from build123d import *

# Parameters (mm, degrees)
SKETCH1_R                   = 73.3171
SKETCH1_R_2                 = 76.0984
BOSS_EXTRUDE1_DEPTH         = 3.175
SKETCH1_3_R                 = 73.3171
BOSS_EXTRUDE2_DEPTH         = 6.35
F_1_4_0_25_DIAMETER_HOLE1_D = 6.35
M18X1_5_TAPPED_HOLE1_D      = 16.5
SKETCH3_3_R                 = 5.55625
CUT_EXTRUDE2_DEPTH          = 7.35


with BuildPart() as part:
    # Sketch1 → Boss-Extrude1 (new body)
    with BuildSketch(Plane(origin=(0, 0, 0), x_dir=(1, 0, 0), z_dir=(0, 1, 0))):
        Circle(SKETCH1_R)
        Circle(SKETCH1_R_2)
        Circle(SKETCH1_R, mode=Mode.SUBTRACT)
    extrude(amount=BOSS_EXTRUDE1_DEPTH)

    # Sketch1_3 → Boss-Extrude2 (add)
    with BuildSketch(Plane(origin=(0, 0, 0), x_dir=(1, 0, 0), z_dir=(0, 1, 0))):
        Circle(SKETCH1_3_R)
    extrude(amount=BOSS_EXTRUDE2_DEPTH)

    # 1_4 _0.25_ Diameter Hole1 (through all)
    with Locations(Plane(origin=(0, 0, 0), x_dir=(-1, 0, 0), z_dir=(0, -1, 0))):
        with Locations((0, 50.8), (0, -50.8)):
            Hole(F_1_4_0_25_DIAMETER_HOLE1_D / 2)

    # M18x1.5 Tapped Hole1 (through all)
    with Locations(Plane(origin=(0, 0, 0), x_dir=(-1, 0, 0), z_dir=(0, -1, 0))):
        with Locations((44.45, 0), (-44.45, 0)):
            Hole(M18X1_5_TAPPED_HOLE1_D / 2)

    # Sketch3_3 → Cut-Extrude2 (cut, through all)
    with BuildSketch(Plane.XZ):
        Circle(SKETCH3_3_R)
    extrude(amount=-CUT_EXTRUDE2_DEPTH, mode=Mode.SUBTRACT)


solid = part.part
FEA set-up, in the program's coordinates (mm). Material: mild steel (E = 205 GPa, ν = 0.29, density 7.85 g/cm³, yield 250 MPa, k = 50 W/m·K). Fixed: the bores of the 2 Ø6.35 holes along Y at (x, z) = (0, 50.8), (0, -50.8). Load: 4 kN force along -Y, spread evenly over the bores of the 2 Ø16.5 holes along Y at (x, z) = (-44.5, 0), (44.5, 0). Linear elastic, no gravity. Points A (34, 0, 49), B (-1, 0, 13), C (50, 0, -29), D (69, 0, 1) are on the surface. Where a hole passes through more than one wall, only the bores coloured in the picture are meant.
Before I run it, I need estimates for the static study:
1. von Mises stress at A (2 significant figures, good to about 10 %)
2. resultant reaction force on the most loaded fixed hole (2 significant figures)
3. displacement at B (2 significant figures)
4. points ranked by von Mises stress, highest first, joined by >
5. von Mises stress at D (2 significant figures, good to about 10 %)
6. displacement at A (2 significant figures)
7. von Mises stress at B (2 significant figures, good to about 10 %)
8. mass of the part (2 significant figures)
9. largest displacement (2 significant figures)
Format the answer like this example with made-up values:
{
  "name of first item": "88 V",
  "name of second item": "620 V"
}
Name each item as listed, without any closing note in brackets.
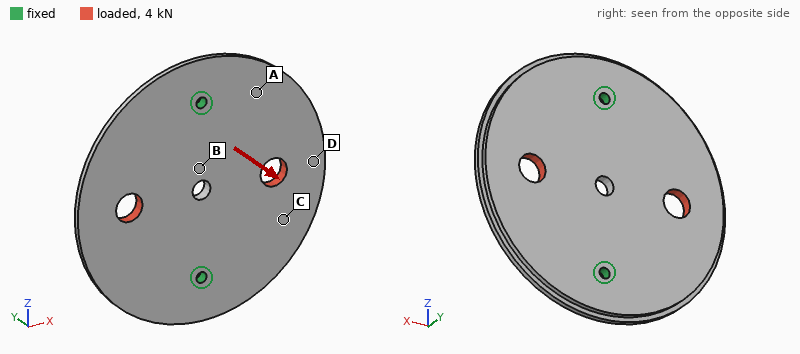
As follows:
{
  "von Mises stress at A": "37 MPa",
  "resultant reaction force on the most loaded fixed hole": "2.0 kN",
  "displacement at B": "0.060 mm",
  "points ranked by von Mises stress, highest first, joined by >": "B > D > A > C",
  "von Mises stress at D": "63 MPa",
  "displacement at A": "0.059 mm",
  "von Mises stress at B": "100 MPa",
  "mass of the part": "850 g",
  "largest displacement": "0.28 mm"
}
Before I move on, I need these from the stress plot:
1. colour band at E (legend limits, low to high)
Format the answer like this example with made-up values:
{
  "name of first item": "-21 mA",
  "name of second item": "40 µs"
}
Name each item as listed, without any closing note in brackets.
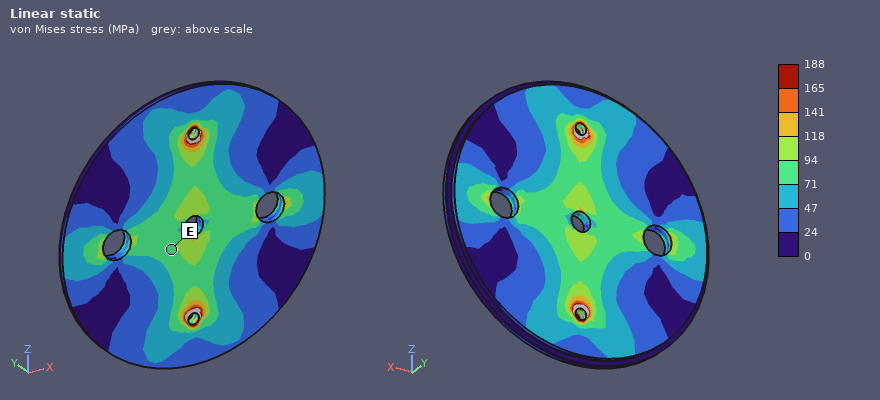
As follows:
{
  "colour band at E": "71 to 94 MPa"
}
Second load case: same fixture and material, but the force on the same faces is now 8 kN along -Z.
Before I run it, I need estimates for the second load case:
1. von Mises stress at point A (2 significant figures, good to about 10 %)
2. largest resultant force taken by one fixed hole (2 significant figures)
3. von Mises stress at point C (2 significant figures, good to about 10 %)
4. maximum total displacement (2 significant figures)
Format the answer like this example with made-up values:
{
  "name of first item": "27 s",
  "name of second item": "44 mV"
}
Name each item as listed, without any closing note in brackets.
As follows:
{
  "von Mises stress at point A": "5.6 MPa",
  "largest resultant force taken by one fixed hole": "4.0 kN",
  "von Mises stress at point C": "6.4 MPa",
  "maximum total displacement": "5.8 µm"
}
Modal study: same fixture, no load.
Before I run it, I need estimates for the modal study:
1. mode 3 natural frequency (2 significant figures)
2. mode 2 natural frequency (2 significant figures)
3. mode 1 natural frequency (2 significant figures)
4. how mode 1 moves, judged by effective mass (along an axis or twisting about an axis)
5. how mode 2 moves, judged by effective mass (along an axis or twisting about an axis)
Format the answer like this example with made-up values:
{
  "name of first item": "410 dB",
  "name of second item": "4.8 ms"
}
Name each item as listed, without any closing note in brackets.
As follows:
{
  "mode 3 natural frequency": "2200 Hz",
  "mode 2 natural frequency": "1100 Hz",
  "mode 1 natural frequency": "860 Hz",
  "how mode 1 moves, judged by effective mass": "twisting about Z",
  "how mode 2 moves, judged by effective mass": "along Y"
}
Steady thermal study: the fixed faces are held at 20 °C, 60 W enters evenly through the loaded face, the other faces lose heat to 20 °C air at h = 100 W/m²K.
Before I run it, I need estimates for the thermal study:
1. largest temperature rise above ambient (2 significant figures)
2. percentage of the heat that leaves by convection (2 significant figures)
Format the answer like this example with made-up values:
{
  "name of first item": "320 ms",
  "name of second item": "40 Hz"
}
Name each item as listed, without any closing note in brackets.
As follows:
{
  "largest temperature rise above ambient": "35 K",
  "percentage of the heat that leaves by convection": "80 %"
}
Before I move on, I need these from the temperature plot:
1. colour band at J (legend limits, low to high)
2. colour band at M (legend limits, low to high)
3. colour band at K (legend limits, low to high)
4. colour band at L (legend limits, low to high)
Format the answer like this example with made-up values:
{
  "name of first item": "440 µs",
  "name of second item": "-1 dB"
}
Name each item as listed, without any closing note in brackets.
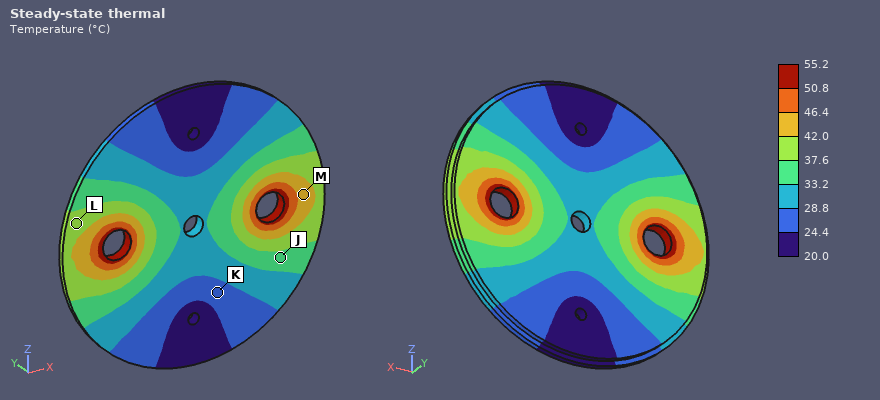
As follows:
{
  "colour band at J": "33.2 to 37.6 °C",
  "colour band at M": "42.0 to 46.4 °C",
  "colour band at K": "24.4 to 28.8 °C",
  "colour band at L": "37.6 to 42.0 °C"
}
